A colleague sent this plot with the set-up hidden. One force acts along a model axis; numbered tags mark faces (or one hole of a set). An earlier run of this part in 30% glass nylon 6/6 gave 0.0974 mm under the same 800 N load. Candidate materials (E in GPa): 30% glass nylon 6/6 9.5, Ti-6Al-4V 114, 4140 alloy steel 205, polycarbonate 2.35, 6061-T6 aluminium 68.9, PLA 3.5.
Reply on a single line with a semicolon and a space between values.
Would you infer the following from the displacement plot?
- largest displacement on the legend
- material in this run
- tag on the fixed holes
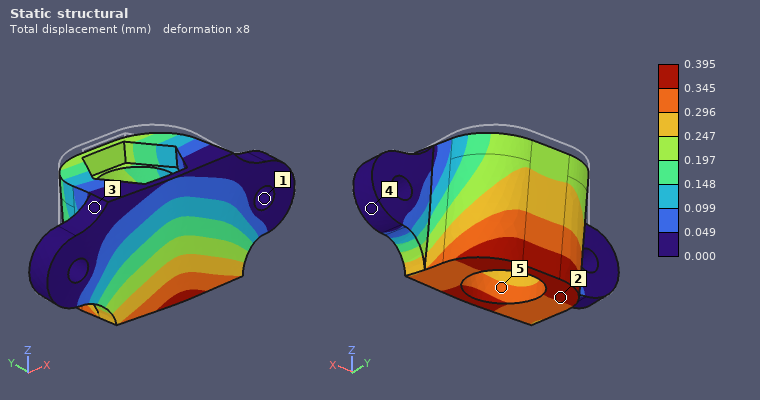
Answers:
0.395 mm; polycarbonate; 1
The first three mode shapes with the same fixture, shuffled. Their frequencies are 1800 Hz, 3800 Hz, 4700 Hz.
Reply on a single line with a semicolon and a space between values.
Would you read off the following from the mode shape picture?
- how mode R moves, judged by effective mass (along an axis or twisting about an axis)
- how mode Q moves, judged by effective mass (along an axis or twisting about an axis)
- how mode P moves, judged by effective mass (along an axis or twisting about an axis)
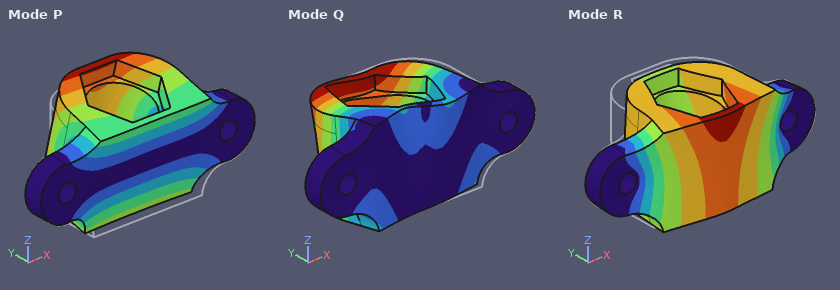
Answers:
along Y; along X; along Z
